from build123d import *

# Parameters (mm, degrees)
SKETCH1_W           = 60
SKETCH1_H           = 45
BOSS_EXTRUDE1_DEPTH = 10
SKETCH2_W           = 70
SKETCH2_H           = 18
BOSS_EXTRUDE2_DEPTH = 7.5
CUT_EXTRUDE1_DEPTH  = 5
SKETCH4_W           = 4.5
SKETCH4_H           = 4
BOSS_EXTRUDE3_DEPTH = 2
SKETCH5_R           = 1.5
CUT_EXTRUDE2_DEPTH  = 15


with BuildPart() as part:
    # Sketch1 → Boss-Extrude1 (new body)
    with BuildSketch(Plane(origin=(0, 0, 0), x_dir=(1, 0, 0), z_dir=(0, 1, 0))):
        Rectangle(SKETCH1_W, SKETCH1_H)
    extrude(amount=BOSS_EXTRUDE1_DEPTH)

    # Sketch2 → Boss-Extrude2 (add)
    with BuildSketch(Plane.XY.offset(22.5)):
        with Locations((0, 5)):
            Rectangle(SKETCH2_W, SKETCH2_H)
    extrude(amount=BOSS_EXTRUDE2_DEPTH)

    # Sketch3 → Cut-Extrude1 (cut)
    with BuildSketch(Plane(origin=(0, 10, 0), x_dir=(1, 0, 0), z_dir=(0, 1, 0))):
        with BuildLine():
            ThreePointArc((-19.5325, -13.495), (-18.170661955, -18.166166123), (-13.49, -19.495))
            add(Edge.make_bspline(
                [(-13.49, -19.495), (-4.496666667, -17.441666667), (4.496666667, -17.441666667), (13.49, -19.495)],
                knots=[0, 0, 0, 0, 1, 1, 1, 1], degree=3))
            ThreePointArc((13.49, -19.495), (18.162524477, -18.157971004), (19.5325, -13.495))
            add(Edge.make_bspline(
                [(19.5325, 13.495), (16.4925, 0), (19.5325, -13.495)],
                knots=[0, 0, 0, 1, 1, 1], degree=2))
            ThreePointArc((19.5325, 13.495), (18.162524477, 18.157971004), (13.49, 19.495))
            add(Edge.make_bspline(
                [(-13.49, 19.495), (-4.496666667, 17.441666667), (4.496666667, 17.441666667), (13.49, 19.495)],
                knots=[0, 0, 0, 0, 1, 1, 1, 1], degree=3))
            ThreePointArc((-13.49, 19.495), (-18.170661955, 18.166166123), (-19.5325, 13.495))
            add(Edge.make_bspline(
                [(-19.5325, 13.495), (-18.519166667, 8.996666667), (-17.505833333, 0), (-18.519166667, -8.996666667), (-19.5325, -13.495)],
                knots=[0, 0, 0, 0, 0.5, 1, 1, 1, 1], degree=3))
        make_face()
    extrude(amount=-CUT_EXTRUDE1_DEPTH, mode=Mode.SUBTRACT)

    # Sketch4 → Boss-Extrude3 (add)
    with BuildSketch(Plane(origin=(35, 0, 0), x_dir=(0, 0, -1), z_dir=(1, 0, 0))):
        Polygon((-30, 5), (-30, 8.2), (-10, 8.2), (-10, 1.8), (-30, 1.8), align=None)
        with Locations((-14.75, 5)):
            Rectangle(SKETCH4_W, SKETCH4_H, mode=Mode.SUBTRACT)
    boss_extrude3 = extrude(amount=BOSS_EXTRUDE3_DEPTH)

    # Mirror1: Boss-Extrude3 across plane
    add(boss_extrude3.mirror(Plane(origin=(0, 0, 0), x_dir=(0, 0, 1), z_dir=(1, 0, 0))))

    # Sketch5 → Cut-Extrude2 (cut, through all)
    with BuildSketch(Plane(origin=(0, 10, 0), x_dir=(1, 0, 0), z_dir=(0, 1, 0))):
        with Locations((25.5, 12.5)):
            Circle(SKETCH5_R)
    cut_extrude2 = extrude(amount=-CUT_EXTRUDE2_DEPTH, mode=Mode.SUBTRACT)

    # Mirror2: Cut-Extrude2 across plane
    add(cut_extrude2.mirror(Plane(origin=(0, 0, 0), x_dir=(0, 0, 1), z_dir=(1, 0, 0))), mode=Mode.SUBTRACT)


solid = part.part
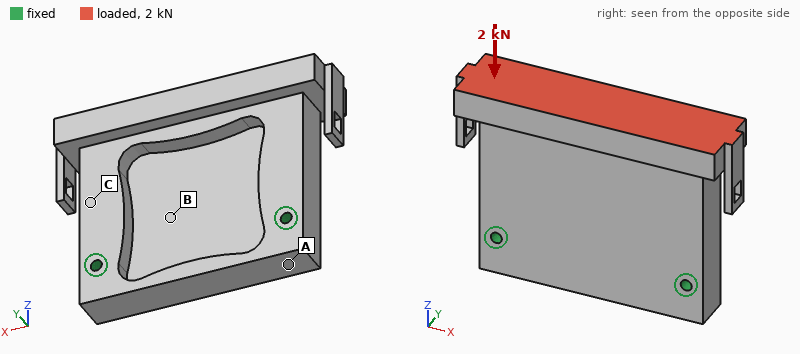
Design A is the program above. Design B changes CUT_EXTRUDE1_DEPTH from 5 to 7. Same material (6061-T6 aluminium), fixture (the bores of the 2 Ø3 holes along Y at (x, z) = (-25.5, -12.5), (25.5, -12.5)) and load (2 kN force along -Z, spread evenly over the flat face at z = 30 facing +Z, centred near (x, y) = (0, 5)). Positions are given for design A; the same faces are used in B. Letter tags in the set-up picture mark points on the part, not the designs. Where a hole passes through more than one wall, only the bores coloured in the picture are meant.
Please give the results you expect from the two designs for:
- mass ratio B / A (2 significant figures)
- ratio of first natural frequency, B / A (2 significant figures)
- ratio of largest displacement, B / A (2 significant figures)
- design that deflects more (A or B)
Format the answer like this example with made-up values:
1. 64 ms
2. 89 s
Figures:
1. 0.91
2. 0.99
3. 1.3
4. B
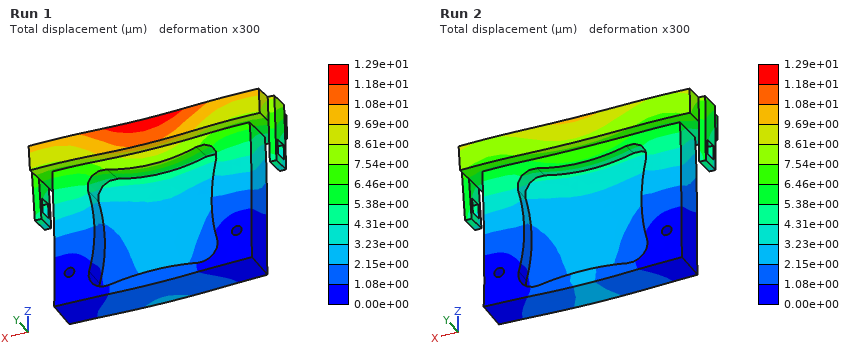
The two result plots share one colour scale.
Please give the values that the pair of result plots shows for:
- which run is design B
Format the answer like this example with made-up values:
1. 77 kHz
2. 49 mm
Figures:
1. Run 1
